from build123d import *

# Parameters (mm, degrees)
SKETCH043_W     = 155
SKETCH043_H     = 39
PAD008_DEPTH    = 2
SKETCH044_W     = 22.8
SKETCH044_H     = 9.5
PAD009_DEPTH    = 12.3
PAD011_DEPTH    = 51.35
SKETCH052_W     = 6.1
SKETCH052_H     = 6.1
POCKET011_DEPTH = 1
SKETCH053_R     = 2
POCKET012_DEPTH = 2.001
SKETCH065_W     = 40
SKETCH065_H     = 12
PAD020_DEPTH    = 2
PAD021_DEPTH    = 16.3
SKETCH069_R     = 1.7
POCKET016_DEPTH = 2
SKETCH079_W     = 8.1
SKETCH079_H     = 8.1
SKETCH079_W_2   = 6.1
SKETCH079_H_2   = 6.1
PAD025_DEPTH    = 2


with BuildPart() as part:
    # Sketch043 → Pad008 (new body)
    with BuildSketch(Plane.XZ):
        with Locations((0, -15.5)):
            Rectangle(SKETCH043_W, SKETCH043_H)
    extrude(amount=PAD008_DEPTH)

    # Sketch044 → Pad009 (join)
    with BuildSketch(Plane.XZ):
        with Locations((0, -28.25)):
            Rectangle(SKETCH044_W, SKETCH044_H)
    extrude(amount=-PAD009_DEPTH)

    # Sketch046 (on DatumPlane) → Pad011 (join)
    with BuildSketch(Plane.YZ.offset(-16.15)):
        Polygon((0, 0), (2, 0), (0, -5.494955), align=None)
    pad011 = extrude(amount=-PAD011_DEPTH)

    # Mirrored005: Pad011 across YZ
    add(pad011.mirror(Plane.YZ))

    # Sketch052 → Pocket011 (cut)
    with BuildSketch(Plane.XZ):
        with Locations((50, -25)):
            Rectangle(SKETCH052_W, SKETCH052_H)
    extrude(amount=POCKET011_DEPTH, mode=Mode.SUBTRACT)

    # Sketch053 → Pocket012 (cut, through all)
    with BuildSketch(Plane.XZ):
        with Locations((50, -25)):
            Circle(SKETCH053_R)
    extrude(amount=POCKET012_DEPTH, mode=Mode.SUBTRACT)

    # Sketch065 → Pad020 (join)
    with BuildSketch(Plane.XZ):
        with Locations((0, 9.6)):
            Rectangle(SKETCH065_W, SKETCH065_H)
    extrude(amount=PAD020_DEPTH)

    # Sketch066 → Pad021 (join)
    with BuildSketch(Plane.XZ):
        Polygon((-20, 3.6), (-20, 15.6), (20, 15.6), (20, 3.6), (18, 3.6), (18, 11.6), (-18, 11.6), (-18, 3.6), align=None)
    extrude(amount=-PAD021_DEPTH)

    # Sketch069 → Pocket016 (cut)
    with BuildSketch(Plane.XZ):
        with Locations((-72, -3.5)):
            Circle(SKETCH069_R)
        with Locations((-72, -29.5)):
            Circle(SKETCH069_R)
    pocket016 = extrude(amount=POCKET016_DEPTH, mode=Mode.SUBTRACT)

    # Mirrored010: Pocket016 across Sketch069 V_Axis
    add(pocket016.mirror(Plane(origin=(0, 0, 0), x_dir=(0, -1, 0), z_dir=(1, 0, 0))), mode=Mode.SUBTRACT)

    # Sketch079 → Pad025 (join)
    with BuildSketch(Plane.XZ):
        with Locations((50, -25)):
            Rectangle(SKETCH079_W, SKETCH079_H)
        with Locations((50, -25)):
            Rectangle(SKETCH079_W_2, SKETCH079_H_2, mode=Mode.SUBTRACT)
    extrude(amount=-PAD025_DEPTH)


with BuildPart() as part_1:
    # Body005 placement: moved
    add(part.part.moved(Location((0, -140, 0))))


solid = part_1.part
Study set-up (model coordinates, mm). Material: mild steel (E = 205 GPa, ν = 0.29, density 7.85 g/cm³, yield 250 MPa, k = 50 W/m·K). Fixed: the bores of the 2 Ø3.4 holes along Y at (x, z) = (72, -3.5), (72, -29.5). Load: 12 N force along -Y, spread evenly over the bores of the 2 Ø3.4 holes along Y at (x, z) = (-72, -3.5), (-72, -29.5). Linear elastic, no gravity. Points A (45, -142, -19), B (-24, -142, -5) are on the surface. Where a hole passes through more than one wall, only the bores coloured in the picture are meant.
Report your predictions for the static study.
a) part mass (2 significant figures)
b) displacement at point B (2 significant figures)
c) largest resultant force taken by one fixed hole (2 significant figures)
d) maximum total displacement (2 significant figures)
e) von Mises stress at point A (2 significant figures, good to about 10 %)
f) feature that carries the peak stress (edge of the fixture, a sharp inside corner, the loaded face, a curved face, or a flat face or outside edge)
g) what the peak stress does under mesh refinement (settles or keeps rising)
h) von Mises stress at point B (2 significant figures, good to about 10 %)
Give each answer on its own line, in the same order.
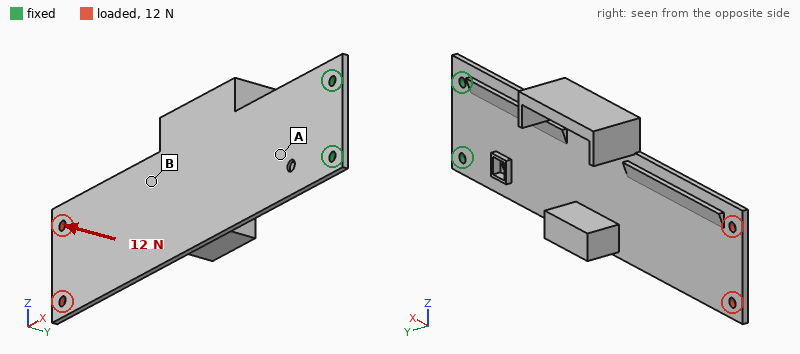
150 g
0.79 mm
19 N
1.5 mm
39 MPa
edge of the fixture
keeps rising
19 MPa
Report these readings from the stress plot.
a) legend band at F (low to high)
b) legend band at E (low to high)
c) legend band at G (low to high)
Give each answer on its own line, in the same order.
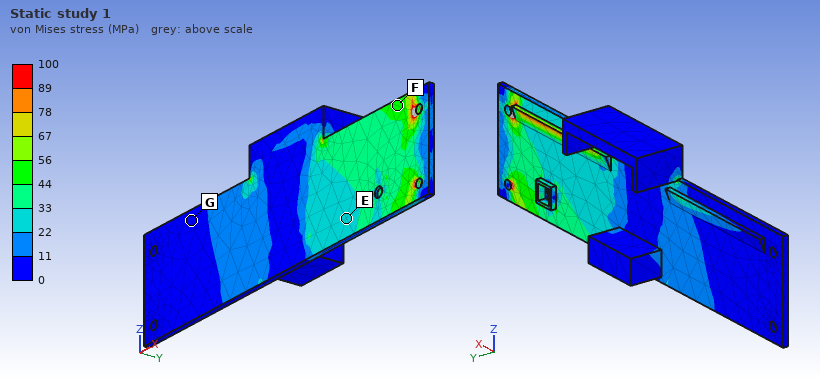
44 to 56 MPa
22 to 33 MPa
0 to 11 MPa
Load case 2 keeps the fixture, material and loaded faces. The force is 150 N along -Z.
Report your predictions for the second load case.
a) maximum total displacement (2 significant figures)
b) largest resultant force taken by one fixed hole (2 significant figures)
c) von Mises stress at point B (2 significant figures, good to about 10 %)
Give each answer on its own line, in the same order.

0.15 mm
800 N
8.3 MPa
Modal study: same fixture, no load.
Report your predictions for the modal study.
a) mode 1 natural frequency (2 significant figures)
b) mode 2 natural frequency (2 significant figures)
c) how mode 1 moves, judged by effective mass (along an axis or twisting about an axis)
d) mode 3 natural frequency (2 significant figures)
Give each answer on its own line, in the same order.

78 Hz
350 Hz
along Y
490 Hz
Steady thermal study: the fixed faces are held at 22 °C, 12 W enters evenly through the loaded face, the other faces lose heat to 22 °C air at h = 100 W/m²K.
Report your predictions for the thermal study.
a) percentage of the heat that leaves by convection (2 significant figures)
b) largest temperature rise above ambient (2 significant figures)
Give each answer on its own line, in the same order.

100 %
67 K
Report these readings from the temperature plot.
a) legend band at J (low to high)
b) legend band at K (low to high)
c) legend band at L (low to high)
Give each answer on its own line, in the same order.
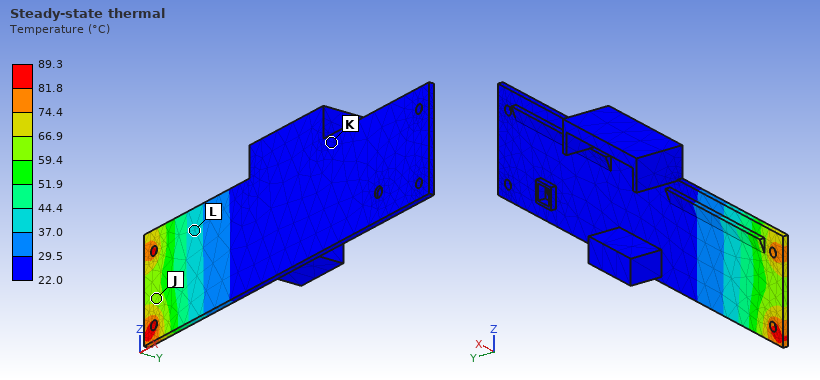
59.4 to 66.9 °C
22.0 to 29.5 °C
37.0 to 44.4 °C
